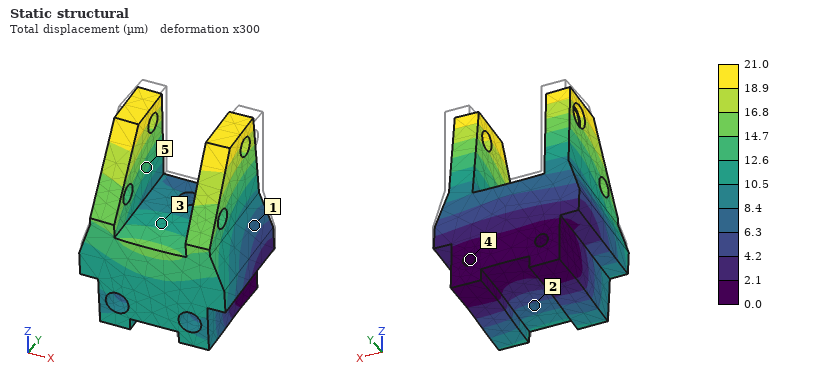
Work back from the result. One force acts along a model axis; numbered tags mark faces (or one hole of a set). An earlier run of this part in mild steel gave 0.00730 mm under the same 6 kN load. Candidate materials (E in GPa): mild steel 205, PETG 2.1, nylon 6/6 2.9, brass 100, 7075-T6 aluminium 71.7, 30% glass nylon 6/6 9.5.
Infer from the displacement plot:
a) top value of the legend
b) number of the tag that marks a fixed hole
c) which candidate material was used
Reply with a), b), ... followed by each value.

a) 21.0 µm
b) 4
c) 7075-T6 aluminium
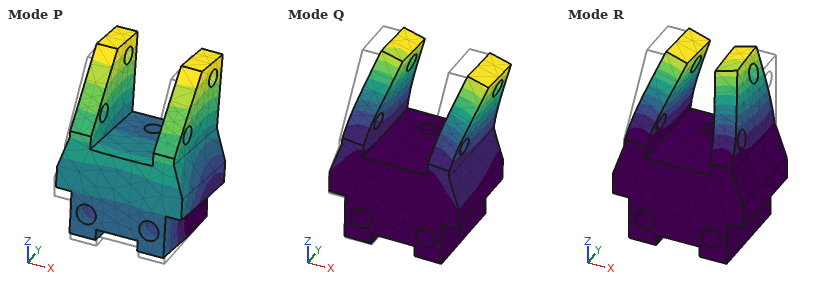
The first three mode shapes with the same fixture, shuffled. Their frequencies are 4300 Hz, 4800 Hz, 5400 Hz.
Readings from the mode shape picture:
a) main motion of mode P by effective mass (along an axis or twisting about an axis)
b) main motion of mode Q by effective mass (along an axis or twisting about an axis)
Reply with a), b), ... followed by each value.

a) along Y
b) along X
